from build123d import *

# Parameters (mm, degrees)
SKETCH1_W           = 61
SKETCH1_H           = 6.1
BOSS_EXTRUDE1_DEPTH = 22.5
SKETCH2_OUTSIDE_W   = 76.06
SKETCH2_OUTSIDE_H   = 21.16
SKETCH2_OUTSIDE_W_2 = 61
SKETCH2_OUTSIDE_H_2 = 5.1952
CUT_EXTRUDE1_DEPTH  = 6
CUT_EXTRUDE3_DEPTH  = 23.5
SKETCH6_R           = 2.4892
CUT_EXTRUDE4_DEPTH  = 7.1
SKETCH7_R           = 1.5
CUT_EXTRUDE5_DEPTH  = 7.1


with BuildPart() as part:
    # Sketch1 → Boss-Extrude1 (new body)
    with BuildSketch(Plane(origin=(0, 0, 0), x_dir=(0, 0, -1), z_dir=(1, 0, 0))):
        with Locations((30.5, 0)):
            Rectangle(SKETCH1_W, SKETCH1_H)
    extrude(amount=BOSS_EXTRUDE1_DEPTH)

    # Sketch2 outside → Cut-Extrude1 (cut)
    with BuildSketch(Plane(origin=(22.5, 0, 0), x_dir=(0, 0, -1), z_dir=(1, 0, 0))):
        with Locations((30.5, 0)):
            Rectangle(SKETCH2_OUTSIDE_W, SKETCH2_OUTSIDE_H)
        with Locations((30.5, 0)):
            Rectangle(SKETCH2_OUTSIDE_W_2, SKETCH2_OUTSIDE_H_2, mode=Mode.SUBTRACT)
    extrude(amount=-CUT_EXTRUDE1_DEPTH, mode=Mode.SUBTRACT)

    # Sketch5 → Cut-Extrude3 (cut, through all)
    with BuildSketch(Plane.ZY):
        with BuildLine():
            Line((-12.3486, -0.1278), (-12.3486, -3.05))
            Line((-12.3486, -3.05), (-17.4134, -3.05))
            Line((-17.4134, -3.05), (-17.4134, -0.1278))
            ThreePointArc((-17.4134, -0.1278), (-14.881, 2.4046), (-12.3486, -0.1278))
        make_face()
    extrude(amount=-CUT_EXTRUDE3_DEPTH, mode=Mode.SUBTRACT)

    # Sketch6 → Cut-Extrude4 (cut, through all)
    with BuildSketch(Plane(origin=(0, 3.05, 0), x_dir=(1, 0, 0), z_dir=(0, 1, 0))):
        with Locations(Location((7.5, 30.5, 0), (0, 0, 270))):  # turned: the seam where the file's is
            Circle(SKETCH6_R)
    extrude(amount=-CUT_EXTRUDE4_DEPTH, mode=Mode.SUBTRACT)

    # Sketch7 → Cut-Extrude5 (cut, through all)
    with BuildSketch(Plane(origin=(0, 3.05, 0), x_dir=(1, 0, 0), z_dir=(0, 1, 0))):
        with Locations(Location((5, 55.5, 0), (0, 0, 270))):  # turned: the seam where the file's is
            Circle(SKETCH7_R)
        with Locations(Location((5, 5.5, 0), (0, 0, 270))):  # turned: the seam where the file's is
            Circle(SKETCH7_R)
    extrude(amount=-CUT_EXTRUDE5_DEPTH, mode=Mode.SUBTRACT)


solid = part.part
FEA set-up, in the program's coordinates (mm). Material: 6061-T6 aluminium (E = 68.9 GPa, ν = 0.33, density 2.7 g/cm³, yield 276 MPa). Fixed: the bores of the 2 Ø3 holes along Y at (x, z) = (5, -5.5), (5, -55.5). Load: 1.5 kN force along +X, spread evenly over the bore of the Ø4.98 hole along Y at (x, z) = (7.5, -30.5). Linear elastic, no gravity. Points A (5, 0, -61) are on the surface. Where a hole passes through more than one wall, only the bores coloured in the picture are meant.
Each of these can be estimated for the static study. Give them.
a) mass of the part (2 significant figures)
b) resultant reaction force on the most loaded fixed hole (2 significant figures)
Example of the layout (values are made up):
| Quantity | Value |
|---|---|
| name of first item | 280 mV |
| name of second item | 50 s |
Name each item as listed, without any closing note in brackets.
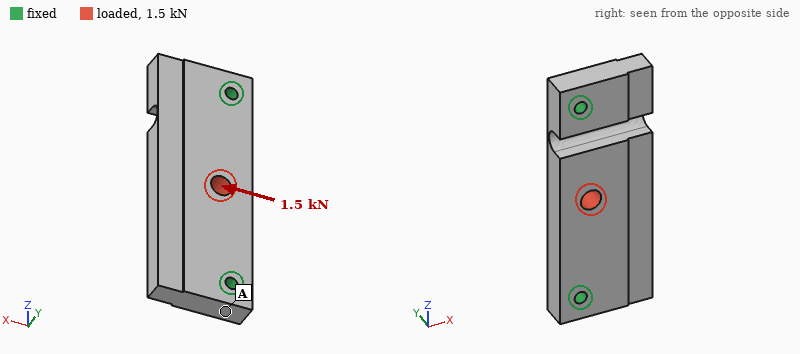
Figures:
| Quantity | Value |
|---|---|
| mass of the part | 20 g |
| resultant reaction force on the most loaded fixed hole | 840 N |
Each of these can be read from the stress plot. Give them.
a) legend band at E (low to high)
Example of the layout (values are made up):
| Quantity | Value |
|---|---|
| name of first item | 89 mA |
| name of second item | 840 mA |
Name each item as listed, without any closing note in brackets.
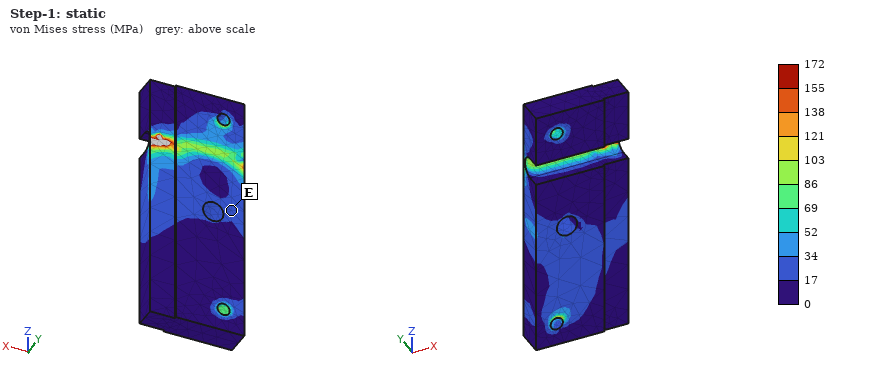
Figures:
| Quantity | Value |
|---|---|
| legend band at E | 17 to 34 MPa |
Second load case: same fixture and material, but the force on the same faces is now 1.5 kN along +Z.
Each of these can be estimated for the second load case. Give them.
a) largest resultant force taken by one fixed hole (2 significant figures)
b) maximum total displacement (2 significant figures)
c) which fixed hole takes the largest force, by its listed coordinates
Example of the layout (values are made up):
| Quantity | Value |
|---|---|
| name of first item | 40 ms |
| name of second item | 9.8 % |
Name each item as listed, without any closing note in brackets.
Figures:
| Quantity | Value |
|---|---|
| largest resultant force taken by one fixed hole | 1.2 kN |
| maximum total displacement | 8.7 µm |
| which fixed hole takes the largest force, by its listed coordinates | (5, -55.5) |
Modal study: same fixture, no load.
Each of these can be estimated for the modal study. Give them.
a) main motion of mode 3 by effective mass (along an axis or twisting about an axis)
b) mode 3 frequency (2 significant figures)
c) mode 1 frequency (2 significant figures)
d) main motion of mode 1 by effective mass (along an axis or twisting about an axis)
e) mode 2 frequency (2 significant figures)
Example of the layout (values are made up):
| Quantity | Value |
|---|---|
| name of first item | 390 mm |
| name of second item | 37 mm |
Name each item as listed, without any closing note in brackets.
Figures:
| Quantity | Value |
|---|---|
| main motion of mode 3 by effective mass | along X |
| mode 3 frequency | 14 kHz |
| mode 1 frequency | 6600 Hz |
| main motion of mode 1 by effective mass | along Y |
| mode 2 frequency | 9900 Hz |
